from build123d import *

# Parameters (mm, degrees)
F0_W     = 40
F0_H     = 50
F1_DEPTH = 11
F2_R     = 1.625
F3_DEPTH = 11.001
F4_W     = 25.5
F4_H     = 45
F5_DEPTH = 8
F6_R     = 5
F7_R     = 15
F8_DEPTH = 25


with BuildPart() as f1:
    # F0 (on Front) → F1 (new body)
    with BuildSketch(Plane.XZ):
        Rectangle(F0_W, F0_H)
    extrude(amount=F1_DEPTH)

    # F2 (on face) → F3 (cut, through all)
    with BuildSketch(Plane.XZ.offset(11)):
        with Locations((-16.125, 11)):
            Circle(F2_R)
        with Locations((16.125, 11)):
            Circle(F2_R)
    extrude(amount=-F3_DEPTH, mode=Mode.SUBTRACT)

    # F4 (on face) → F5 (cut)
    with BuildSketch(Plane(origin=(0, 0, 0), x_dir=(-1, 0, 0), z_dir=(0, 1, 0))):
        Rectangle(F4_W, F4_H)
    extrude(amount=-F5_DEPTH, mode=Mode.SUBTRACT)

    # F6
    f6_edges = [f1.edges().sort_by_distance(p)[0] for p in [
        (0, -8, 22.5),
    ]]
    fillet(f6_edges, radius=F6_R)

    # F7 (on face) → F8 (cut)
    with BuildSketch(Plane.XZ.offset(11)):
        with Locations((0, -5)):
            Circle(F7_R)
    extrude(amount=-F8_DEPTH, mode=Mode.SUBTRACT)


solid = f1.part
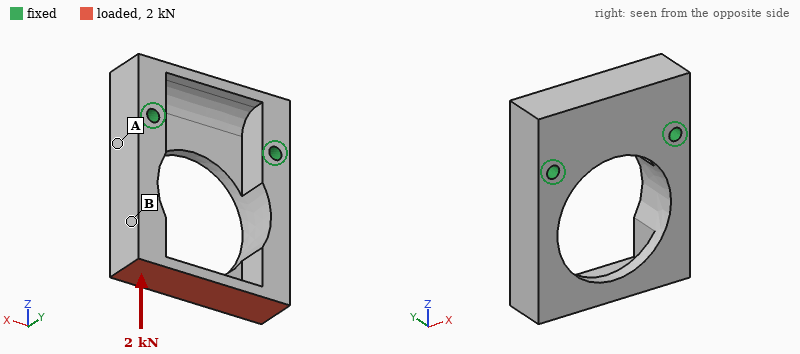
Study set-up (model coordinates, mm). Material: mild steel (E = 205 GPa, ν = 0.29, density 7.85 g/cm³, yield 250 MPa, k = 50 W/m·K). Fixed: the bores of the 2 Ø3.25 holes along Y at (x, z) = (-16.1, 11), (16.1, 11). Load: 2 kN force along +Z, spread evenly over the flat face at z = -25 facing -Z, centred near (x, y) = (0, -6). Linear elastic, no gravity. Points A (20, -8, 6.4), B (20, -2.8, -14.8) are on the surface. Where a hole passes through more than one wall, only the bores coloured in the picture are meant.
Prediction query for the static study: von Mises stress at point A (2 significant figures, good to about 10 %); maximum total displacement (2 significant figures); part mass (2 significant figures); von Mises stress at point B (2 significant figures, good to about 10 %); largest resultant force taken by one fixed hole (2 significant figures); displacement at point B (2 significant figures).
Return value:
35 MPa
26 µm
81 g
12 MPa
1.1 kN
4.1 µm
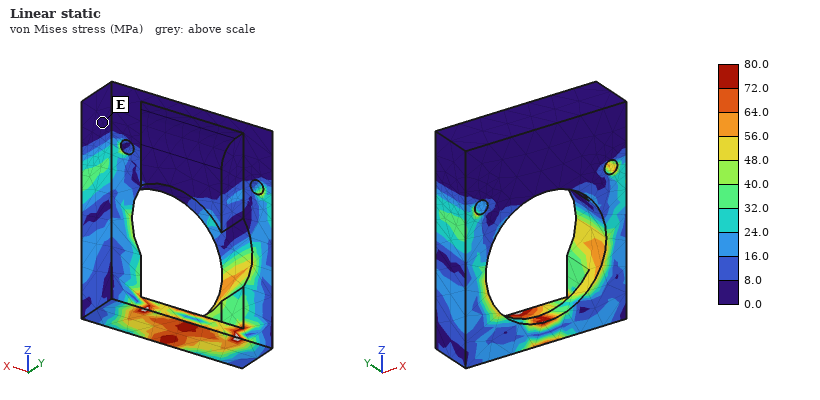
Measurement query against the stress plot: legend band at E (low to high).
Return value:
0.0 to 8.0 MPa
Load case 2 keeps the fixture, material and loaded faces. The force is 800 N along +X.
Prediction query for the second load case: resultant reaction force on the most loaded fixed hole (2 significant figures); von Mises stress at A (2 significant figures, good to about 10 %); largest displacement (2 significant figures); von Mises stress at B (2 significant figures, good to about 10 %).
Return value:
720 N
63 MPa
36 µm
19 MPa
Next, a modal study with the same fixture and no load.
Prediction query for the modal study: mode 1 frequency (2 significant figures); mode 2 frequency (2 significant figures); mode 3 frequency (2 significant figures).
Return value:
5100 Hz
5200 Hz
8000 Hz
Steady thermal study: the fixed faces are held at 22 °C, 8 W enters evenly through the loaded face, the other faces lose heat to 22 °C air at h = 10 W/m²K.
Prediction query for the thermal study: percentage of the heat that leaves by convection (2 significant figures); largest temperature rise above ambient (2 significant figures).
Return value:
8.6 %
44 K
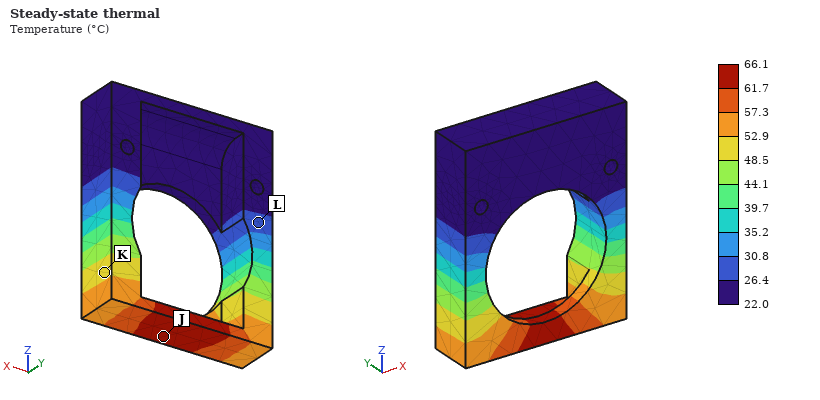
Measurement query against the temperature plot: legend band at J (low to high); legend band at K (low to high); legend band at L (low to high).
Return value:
61.7 to 66.1 °C
48.5 to 52.9 °C
26.4 to 30.8 °C
